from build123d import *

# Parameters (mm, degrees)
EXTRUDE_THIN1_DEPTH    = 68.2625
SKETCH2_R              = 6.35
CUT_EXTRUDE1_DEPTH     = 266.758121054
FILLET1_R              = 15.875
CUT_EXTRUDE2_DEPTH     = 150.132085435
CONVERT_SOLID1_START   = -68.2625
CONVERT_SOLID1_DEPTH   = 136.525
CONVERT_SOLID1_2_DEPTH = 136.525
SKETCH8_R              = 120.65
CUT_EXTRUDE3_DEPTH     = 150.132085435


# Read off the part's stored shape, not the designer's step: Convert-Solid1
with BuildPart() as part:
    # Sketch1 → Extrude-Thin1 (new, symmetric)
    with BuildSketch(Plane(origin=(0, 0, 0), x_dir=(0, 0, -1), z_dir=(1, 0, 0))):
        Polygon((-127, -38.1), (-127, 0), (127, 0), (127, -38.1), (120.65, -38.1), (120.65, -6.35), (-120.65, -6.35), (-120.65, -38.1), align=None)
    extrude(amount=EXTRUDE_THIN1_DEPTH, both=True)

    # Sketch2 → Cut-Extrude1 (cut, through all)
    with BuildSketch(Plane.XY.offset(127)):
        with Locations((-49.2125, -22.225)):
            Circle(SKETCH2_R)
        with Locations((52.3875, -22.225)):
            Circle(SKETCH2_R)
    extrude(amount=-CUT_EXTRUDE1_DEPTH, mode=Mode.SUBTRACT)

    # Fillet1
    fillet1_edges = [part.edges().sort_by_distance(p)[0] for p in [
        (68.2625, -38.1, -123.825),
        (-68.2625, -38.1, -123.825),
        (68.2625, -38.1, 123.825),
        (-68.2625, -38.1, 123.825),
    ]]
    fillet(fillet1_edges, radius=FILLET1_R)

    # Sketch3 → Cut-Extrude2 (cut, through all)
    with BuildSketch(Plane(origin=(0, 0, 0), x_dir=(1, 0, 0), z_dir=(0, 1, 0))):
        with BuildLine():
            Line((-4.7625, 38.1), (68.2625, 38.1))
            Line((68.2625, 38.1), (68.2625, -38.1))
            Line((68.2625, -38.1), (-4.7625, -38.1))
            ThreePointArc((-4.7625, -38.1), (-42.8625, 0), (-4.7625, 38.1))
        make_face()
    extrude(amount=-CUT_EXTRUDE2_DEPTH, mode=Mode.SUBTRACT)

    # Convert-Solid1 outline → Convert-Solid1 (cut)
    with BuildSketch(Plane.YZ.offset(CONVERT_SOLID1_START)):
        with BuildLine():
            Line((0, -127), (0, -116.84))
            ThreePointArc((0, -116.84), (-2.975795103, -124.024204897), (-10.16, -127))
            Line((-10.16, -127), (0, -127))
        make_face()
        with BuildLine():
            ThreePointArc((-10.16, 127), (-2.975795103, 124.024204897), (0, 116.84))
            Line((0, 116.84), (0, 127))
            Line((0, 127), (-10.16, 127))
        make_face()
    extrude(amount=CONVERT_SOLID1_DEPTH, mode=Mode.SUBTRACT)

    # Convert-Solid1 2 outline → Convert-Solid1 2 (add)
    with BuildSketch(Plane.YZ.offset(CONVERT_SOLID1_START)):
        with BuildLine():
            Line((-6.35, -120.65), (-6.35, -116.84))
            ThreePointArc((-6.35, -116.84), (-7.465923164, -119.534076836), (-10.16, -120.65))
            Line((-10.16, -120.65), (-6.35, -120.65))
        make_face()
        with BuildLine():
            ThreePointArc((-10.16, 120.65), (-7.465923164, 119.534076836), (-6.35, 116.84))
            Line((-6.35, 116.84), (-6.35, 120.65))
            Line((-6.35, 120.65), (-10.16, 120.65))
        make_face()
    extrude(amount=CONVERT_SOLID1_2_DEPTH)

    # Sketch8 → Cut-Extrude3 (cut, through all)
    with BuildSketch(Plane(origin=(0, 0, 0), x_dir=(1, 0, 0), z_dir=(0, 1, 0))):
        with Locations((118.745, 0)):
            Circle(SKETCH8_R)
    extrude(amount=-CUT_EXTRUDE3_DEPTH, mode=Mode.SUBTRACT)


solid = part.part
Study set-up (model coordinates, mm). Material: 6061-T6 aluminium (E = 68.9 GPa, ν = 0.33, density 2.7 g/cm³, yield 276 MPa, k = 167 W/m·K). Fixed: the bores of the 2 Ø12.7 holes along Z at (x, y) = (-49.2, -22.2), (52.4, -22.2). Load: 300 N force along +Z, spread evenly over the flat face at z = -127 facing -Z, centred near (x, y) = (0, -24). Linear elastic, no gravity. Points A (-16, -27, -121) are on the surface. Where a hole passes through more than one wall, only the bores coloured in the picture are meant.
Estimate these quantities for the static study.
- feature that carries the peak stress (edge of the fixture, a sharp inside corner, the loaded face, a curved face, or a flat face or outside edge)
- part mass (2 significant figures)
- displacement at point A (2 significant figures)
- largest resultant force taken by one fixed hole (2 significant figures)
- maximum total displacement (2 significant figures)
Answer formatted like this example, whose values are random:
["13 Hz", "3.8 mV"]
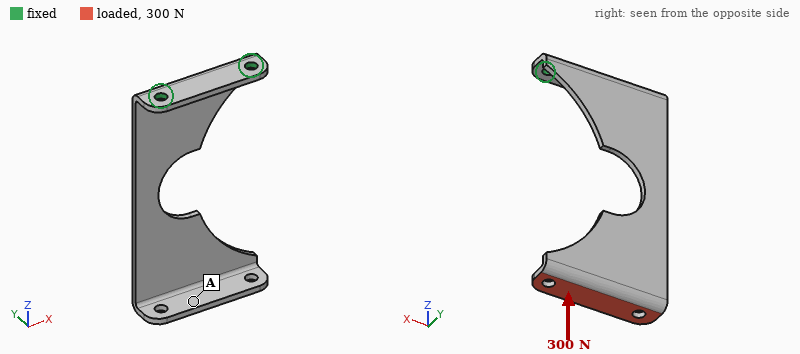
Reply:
["a curved face", "480 g", "2.6 mm", "170 N", "2.8 mm"]
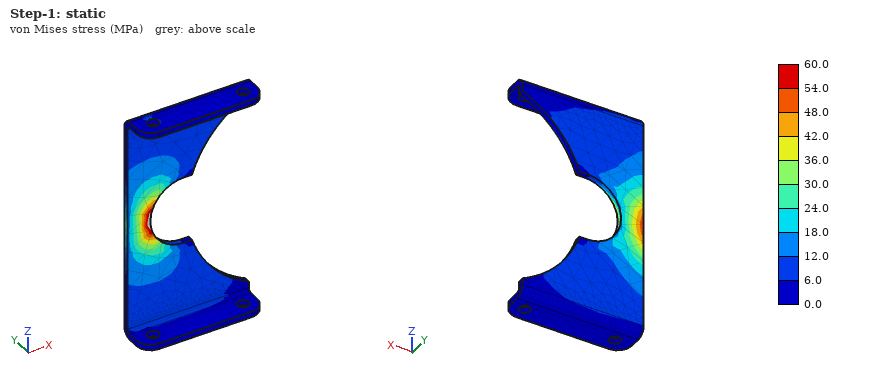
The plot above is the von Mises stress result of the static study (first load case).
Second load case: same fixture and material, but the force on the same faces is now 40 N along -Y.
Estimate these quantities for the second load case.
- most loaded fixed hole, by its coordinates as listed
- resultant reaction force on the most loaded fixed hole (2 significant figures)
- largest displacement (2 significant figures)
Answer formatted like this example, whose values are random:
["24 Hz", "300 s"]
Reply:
["(-49.2, -22.2)", "23 N", "3.2 mm"]
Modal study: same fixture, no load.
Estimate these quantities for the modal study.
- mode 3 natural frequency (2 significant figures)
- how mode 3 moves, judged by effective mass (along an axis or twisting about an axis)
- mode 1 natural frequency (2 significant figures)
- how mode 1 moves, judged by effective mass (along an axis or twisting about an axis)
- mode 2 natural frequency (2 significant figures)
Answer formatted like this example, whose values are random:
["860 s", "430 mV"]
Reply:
["280 Hz", "along X", "47 Hz", "along Y", "190 Hz"]
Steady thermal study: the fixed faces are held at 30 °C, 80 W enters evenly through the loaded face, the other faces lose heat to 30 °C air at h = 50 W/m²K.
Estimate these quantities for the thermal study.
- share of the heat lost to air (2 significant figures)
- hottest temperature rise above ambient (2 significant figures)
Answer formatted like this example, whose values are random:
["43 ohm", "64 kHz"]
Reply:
["94 %", "73 K"]
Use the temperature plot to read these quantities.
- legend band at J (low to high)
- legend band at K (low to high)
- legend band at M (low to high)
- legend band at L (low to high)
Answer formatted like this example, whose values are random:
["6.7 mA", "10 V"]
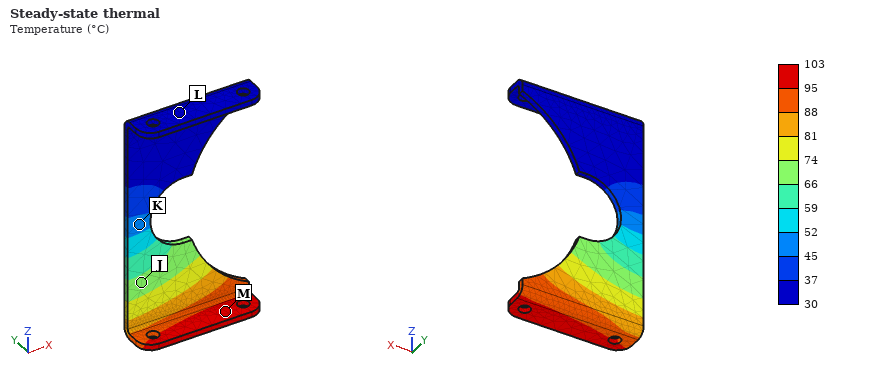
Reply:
["66 to 74 °C", "45 to 52 °C", "95 to 103 °C", "30 to 37 °C"]
